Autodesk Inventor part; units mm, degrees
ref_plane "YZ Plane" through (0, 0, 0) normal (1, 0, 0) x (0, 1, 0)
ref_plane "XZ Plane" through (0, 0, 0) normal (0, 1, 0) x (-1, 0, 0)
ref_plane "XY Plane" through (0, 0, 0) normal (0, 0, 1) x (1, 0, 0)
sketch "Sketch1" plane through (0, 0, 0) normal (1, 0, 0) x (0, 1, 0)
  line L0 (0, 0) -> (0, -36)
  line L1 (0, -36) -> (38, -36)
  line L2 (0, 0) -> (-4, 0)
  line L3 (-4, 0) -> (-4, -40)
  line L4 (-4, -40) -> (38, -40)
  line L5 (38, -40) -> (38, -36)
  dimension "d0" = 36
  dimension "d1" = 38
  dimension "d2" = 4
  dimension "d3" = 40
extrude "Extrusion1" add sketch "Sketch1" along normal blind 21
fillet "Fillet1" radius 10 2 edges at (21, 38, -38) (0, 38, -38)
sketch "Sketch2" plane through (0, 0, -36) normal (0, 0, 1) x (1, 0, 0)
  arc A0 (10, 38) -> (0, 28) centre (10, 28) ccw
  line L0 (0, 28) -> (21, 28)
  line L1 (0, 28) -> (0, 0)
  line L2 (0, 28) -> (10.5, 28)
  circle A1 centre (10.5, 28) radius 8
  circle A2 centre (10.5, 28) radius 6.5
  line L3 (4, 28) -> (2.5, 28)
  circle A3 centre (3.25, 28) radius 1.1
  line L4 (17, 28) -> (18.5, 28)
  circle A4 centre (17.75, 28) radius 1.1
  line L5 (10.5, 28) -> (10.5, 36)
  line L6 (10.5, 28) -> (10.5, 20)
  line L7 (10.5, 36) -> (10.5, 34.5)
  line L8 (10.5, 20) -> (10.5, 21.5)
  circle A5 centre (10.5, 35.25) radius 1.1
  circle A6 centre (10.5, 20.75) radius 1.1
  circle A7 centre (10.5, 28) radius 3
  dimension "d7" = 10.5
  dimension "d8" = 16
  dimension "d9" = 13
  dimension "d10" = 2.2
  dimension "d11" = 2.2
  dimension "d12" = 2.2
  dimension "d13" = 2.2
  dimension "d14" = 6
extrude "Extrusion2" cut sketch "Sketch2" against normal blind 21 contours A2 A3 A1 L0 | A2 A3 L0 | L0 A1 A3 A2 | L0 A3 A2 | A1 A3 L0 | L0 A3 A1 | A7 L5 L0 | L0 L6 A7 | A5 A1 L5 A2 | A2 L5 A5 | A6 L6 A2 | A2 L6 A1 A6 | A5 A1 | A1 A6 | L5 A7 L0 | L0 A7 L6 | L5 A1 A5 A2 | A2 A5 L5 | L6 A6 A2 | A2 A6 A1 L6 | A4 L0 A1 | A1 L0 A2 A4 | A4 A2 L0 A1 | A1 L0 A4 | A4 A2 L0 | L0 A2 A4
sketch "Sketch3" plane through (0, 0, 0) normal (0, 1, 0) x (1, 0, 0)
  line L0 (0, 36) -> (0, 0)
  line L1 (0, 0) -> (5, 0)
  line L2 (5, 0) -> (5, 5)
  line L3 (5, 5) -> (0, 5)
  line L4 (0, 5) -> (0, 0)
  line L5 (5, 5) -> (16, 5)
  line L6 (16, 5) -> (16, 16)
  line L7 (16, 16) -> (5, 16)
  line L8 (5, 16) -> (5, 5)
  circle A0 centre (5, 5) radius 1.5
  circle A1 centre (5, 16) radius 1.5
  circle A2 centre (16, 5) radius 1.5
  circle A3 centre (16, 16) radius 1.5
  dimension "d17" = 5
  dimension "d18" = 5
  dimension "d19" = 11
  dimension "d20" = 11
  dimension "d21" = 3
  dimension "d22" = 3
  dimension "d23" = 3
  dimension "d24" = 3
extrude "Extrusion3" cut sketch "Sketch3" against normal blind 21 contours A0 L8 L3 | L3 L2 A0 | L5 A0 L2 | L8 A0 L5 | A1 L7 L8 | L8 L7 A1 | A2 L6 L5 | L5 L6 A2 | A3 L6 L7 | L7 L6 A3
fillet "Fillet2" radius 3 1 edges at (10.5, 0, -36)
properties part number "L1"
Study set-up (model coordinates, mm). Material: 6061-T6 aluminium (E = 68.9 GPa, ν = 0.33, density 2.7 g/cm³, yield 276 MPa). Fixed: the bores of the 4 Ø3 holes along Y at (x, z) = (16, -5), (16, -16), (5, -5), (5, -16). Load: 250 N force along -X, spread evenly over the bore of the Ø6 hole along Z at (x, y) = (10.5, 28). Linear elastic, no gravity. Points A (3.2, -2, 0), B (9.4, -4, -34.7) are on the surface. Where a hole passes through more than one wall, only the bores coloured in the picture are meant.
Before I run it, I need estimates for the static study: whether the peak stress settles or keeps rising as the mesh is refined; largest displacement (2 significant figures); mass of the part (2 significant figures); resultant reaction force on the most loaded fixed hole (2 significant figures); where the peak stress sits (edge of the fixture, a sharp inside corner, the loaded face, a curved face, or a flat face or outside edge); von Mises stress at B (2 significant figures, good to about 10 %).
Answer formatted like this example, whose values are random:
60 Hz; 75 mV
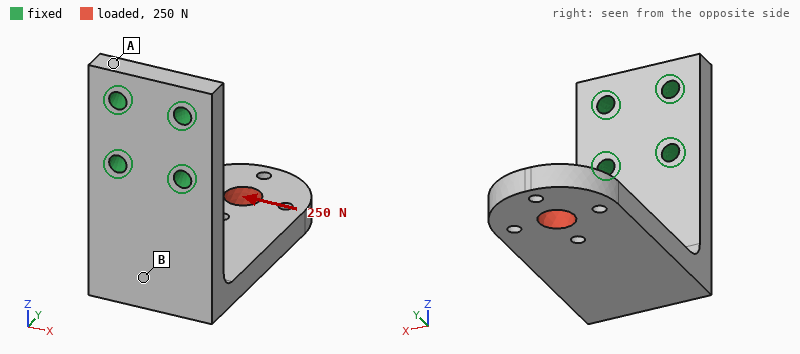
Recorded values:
keeps rising; 0.41 mm; 17 g; 650 N; edge of the fixture; 70 MPa
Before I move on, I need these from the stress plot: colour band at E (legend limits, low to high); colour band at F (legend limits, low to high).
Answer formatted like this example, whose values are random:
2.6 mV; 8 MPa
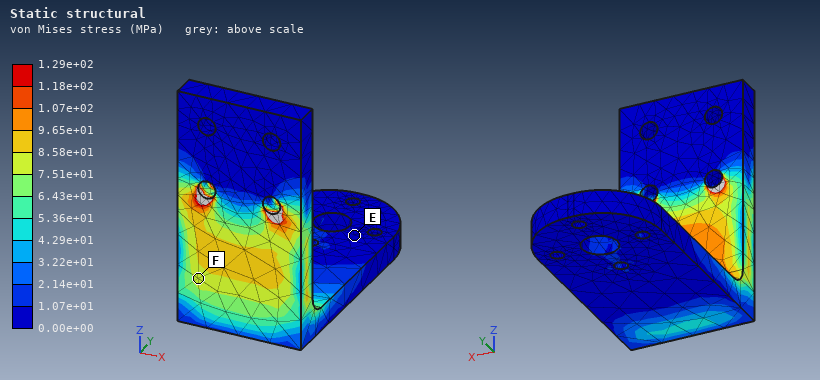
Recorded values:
0.00e+00 to 1.07e+01 MPa; 7.51e+01 to 8.58e+01 MPa
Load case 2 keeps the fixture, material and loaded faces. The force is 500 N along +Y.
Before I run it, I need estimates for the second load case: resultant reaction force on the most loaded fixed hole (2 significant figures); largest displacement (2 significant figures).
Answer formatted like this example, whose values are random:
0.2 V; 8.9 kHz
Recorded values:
350 N; 0.63 mm
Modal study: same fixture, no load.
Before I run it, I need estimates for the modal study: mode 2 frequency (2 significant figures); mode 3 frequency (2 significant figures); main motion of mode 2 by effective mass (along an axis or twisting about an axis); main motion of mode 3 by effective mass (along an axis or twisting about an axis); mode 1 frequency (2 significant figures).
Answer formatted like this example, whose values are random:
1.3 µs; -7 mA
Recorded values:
2100 Hz; 4100 Hz; along X; along Y; 1300 Hz
